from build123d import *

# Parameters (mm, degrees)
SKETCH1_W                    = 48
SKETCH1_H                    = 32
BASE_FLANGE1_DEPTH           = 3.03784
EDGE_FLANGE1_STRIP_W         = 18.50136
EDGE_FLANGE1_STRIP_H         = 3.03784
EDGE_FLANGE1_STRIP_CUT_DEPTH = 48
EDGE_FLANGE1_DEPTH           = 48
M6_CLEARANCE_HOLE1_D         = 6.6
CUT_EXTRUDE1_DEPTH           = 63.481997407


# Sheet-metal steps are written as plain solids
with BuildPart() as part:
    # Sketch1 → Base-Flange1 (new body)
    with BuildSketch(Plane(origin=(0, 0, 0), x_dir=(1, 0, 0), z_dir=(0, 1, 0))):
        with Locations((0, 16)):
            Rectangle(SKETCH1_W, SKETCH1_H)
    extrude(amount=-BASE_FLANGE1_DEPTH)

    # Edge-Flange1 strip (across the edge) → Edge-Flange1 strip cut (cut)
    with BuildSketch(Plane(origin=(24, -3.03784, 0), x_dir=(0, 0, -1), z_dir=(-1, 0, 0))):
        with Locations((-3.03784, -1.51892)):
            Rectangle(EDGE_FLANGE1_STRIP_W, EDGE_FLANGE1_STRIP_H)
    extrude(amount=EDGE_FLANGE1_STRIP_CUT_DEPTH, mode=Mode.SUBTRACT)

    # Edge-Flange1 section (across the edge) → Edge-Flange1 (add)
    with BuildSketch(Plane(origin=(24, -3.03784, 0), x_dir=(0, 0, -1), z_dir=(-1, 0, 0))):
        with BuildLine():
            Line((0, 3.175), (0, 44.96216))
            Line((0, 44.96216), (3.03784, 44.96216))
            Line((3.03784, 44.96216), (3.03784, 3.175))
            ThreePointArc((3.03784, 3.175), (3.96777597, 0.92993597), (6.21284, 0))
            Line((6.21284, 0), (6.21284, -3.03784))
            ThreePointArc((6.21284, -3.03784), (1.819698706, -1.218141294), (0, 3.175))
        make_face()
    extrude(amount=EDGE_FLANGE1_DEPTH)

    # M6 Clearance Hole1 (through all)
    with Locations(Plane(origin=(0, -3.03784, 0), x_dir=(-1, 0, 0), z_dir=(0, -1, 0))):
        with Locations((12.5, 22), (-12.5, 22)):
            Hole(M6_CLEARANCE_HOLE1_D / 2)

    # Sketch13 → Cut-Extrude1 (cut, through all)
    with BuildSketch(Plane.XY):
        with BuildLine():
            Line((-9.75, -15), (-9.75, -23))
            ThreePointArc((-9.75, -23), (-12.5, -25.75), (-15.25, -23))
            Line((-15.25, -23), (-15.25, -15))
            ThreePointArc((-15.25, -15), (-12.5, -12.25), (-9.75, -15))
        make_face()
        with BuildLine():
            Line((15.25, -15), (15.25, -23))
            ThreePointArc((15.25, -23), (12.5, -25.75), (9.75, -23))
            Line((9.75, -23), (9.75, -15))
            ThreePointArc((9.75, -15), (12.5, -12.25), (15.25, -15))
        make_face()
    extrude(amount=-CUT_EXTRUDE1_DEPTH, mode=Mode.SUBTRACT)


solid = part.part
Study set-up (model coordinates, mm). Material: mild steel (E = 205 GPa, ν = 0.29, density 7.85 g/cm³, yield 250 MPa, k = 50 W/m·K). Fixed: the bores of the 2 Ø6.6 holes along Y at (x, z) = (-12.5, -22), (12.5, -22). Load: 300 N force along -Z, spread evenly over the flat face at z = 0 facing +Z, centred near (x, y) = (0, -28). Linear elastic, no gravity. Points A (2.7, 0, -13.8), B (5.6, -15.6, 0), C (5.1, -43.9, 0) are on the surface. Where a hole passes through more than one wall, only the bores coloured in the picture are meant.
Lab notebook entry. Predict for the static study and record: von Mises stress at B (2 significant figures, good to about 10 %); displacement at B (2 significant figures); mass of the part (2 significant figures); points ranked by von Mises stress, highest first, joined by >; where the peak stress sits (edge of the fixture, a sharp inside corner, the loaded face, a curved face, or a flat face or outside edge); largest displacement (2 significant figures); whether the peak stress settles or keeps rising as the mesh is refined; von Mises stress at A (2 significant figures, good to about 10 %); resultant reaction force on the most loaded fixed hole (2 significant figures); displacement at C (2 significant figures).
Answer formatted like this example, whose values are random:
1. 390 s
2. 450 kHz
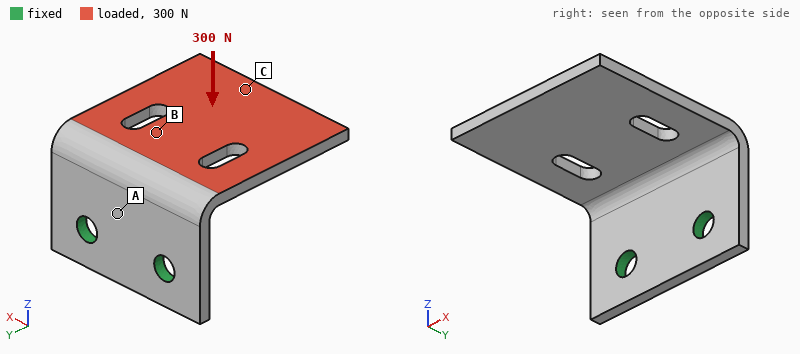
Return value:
1. 65 MPa
2. 0.13 mm
3. 81 g
4. A > B > C
5. edge of the fixture
6. 0.46 mm
7. keeps rising
8. 88 MPa
9. 150 N
10. 0.41 mm
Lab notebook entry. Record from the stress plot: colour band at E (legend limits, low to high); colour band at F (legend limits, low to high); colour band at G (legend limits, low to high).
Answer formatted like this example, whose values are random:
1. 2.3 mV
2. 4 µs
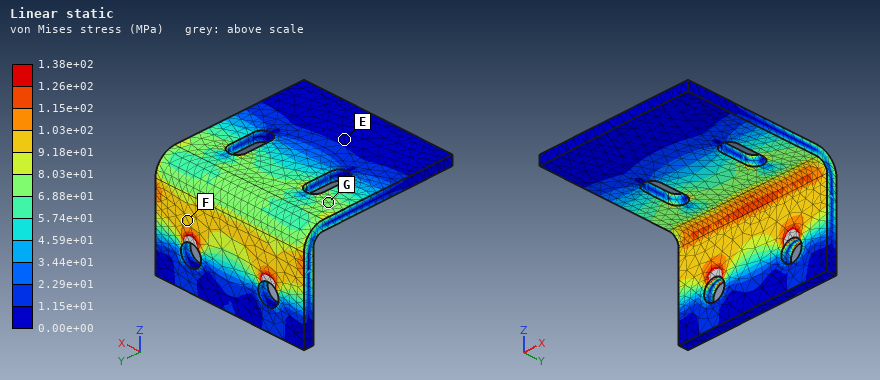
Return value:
1. 0.00e+00 to 1.15e+01 MPa
2. 9.18e+01 to 1.03e+02 MPa
3. 6.88e+01 to 8.03e+01 MPa
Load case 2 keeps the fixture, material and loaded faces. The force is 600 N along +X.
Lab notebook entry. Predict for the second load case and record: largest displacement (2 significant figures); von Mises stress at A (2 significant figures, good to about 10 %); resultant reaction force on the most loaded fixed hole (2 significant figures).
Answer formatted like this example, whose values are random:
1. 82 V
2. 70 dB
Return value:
1. 0.16 mm
2. 54 MPa
3. 720 N
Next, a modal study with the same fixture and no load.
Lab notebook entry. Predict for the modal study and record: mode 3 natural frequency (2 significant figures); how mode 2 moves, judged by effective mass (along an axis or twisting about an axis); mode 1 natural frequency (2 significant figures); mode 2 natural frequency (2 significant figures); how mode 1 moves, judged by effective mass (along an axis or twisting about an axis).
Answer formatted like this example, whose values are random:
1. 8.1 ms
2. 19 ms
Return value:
1. 2600 Hz
2. along X
3. 730 Hz
4. 1600 Hz
5. along Z
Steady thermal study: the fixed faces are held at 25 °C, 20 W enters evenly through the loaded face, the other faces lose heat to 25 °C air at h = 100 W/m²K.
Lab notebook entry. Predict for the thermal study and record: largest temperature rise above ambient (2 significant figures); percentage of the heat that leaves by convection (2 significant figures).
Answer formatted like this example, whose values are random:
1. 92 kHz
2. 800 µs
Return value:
1. 52 K
2. 67 %
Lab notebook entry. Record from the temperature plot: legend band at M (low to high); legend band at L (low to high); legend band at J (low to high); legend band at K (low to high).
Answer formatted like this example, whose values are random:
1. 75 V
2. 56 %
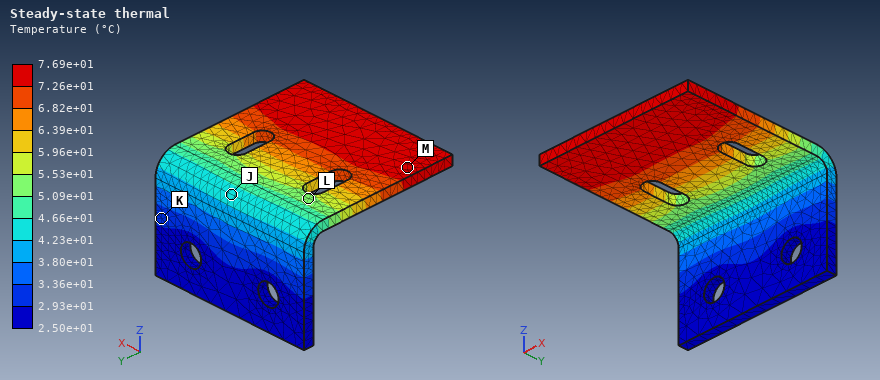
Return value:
1. 7.26e+01 to 7.69e+01 °C
2. 5.09e+01 to 5.53e+01 °C
3. 4.23e+01 to 4.66e+01 °C
4. 2.93e+01 to 3.36e+01 °C
